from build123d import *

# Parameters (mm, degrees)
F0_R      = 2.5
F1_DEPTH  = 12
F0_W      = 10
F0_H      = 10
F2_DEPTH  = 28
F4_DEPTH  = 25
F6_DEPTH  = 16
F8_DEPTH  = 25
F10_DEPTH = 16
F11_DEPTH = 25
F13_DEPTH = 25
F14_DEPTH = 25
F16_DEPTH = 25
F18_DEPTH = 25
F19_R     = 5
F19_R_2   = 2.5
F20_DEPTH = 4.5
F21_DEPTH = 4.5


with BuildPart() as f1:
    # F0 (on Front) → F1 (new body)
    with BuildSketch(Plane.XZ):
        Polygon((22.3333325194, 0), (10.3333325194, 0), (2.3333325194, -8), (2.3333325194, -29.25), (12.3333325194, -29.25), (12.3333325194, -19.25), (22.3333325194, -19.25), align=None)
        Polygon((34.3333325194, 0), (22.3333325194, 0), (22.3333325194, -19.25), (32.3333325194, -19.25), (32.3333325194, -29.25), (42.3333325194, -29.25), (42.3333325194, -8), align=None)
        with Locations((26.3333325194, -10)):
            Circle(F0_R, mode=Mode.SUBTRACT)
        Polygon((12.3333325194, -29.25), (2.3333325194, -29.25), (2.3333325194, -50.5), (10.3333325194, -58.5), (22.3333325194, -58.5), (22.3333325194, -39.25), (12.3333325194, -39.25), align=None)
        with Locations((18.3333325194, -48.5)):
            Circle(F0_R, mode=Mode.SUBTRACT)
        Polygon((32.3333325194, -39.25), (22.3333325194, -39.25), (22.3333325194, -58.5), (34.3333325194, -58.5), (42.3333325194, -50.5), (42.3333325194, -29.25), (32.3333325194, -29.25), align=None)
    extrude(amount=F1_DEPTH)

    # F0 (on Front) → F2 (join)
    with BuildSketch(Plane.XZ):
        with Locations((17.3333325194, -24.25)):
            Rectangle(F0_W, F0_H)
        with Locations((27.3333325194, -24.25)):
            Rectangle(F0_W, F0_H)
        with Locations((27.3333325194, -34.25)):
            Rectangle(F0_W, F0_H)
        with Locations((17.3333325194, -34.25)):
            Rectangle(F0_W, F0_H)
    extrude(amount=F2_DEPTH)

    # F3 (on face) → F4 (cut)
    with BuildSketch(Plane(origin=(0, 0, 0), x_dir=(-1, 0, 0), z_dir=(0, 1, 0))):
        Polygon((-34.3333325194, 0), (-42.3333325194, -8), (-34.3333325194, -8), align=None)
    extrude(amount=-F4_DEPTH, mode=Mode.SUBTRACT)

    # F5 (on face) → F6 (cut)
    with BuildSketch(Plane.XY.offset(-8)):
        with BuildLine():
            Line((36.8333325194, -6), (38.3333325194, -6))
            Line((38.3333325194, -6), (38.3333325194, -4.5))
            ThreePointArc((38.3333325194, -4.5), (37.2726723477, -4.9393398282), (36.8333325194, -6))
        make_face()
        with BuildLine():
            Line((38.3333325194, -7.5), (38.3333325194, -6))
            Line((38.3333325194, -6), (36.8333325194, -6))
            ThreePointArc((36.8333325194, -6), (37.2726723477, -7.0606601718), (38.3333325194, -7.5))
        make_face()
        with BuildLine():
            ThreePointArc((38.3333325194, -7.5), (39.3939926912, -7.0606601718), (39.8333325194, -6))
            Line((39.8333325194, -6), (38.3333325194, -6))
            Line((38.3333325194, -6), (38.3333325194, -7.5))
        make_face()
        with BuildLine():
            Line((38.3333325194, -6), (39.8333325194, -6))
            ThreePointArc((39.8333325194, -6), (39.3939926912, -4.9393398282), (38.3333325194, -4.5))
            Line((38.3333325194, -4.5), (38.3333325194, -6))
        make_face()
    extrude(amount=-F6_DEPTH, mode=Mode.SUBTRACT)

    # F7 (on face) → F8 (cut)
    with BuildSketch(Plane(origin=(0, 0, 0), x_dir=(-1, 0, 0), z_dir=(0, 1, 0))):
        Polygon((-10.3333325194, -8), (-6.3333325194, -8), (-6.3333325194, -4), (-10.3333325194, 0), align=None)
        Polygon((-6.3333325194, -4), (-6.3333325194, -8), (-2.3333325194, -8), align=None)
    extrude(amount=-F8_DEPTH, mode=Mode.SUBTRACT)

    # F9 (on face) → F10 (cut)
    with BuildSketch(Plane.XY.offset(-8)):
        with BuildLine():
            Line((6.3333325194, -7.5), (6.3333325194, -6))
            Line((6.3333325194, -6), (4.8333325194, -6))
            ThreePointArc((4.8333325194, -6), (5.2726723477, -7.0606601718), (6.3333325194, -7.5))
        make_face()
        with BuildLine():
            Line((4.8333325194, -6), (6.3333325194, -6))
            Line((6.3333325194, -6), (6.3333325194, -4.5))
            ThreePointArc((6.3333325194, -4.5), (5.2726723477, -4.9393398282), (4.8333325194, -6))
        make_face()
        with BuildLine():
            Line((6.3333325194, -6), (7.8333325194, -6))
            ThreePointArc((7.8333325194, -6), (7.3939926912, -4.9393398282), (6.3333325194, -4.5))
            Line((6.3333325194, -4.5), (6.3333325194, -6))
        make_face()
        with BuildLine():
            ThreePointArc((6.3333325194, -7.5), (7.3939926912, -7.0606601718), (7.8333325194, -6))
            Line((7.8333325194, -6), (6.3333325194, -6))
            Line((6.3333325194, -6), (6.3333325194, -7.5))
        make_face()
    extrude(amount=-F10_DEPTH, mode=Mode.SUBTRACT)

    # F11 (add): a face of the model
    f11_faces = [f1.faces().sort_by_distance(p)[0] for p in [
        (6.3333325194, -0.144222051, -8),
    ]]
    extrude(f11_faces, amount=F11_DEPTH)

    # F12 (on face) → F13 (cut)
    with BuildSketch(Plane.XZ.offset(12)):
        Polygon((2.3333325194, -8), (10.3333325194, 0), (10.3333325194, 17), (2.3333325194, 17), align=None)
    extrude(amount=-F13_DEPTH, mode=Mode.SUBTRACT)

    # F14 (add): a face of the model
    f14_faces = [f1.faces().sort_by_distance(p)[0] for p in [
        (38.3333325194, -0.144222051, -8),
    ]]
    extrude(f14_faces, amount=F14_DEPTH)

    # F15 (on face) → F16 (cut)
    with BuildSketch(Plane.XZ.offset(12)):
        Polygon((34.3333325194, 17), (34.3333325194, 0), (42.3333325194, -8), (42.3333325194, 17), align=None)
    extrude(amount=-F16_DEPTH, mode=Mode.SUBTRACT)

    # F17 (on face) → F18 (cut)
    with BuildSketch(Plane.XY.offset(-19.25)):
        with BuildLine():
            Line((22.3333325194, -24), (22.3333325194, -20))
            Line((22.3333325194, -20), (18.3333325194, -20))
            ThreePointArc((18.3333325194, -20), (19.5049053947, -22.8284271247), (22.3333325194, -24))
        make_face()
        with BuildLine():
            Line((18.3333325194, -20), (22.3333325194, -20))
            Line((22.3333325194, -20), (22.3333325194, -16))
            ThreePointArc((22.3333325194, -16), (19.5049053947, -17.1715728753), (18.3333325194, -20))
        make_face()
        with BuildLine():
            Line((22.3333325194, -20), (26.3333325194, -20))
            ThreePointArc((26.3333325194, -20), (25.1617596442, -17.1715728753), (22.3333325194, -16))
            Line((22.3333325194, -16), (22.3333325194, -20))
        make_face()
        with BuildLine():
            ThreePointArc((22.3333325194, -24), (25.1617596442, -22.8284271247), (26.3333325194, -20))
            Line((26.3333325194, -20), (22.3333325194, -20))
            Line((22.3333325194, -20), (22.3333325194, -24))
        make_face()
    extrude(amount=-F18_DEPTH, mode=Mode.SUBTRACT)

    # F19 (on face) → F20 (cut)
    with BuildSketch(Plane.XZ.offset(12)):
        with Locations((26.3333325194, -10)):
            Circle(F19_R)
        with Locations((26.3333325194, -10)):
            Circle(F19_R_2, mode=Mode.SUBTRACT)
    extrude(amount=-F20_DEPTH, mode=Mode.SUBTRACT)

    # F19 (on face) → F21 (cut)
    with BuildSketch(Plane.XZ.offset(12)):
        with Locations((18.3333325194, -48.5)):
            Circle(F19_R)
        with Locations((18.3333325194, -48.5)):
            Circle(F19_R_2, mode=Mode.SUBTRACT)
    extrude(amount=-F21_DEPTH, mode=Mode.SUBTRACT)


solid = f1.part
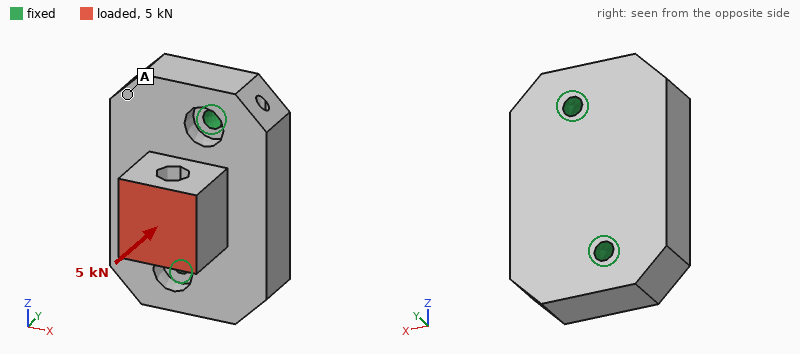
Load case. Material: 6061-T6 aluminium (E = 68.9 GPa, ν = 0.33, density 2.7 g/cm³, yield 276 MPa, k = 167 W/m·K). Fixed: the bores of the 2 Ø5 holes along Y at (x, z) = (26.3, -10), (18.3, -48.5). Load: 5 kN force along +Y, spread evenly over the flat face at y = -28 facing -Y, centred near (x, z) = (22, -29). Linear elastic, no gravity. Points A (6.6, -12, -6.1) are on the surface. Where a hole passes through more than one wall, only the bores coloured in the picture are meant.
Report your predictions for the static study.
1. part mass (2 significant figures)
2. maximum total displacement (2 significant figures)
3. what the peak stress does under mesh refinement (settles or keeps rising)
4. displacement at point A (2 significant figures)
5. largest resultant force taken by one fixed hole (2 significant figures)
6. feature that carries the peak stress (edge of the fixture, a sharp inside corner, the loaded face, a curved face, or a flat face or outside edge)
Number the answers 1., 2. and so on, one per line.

1. 83 g
2. 17 µm
3. keeps rising
4. 7.0 µm
5. 2.7 kN
6. edge of the fixture
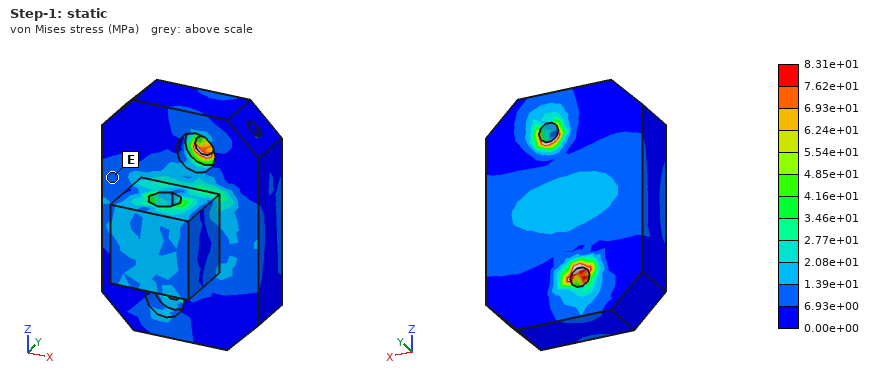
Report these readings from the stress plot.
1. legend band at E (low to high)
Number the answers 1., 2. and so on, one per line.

1. 6.93e+00 to 1.39e+01 MPa
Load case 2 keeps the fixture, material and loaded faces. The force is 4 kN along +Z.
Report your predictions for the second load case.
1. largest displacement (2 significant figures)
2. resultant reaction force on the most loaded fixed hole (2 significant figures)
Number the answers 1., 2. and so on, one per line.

1. 45 µm
2. 3.2 kN
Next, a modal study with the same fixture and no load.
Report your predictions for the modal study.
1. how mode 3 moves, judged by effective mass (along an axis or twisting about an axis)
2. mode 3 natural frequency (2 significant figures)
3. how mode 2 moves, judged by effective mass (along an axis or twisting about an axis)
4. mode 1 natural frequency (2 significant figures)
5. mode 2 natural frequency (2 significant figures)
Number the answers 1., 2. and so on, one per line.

1. along Z
2. 19 kHz
3. along Y
4. 7100 Hz
5. 14 kHz
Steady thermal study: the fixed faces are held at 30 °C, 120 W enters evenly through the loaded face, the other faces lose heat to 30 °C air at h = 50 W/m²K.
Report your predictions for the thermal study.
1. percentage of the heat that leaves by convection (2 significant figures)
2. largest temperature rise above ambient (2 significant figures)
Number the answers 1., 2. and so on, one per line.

1. 5.9 %
2. 62 K
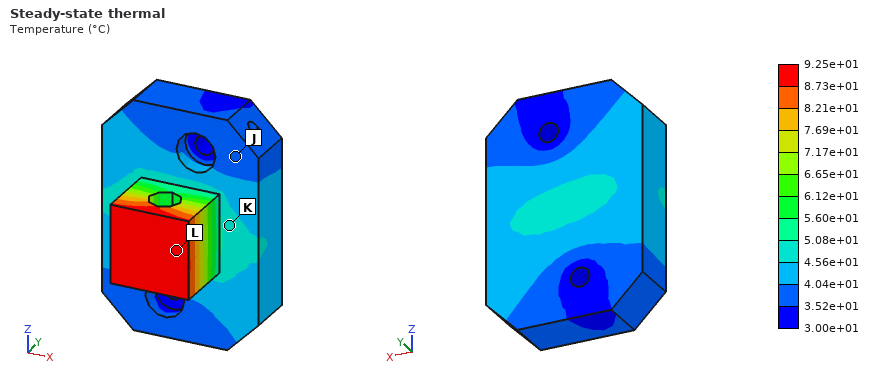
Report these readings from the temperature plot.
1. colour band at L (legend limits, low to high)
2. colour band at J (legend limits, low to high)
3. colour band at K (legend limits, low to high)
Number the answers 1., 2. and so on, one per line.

1. 8.73e+01 to 9.25e+01 °C
2. 3.52e+01 to 4.04e+01 °C
3. 4.56e+01 to 5.08e+01 °C
